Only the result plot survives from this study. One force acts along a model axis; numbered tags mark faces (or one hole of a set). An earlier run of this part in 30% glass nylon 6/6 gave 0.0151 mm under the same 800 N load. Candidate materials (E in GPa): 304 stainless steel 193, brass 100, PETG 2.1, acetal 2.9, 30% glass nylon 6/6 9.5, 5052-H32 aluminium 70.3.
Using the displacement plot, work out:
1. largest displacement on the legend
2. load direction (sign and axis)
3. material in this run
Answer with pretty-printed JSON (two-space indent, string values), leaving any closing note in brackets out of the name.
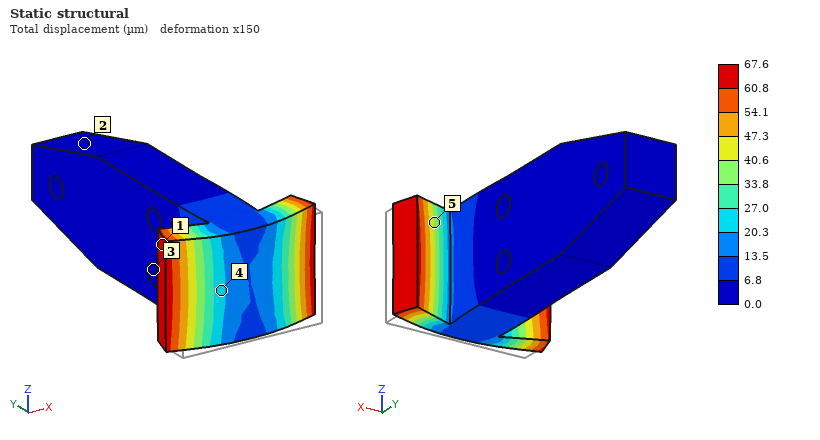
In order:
{
  "largest displacement on the legend": "67.6 µm",
  "load direction": "+Y",
  "material in this run": "PETG"
}
